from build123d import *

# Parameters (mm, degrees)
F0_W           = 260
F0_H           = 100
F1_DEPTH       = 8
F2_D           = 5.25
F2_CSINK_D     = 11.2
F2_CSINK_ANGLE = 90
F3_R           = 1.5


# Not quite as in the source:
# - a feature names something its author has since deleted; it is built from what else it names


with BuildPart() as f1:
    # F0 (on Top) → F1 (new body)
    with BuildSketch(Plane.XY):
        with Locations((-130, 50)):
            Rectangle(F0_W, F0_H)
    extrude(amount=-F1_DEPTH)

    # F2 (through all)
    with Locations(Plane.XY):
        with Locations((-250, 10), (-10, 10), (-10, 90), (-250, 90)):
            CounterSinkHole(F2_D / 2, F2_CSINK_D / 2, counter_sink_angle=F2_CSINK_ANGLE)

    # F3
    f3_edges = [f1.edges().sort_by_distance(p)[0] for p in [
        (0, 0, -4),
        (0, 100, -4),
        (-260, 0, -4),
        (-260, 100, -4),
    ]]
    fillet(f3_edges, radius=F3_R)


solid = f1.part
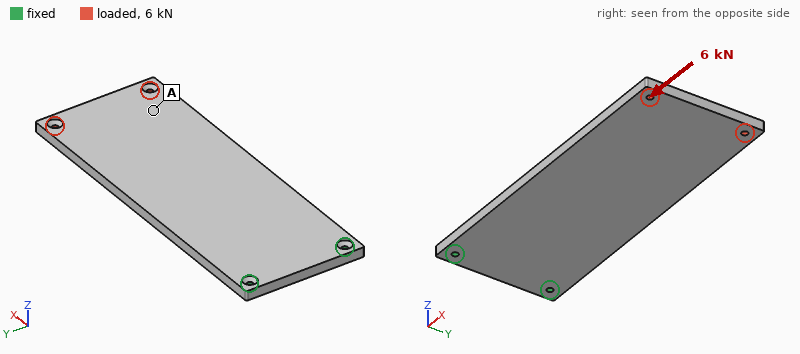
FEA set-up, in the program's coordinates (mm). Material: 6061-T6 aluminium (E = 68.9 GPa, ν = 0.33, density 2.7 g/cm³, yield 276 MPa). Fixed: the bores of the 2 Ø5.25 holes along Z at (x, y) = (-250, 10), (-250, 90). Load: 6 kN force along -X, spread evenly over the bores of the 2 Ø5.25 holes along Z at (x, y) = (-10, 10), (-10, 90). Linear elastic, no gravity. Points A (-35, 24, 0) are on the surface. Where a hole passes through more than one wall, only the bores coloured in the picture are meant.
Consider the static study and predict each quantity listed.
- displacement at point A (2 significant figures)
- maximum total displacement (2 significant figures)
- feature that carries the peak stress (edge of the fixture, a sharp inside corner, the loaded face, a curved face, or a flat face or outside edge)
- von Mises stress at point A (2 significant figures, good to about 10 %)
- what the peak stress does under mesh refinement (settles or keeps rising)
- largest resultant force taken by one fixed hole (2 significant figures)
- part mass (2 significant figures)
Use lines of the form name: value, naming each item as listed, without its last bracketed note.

displacement at point A: 0.74 mm
maximum total displacement: 0.99 mm
feature that carries the peak stress: edge of the fixture
von Mises stress at point A: 4.7 MPa
what the peak stress does under mesh refinement: keeps rising
largest resultant force taken by one fixed hole: 3.1 kN
part mass: 560 g
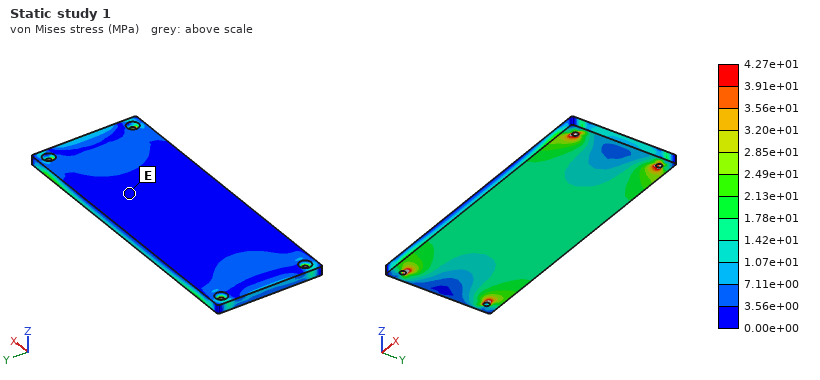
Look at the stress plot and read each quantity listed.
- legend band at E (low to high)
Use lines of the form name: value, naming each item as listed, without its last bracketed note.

legend band at E: 0.00e+00 to 3.56e+00 MPa
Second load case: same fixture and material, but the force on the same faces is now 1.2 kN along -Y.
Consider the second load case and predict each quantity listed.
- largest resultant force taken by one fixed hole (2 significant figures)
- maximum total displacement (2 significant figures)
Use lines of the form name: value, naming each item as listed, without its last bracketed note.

largest resultant force taken by one fixed hole: 3.6 kN
maximum total displacement: 0.18 mm
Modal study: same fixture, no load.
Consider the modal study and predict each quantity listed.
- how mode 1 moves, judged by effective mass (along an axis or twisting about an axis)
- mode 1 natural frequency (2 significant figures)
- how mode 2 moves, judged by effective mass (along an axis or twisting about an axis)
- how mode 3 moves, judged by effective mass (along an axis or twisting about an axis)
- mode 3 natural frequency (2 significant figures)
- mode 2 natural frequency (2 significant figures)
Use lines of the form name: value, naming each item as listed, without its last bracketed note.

how mode 1 moves, judged by effective mass: along Z
mode 1 natural frequency: 91 Hz
how mode 2 moves, judged by effective mass: twisting about X
how mode 3 moves, judged by effective mass: along Z
mode 3 natural frequency: 590 Hz
mode 2 natural frequency: 530 Hz
